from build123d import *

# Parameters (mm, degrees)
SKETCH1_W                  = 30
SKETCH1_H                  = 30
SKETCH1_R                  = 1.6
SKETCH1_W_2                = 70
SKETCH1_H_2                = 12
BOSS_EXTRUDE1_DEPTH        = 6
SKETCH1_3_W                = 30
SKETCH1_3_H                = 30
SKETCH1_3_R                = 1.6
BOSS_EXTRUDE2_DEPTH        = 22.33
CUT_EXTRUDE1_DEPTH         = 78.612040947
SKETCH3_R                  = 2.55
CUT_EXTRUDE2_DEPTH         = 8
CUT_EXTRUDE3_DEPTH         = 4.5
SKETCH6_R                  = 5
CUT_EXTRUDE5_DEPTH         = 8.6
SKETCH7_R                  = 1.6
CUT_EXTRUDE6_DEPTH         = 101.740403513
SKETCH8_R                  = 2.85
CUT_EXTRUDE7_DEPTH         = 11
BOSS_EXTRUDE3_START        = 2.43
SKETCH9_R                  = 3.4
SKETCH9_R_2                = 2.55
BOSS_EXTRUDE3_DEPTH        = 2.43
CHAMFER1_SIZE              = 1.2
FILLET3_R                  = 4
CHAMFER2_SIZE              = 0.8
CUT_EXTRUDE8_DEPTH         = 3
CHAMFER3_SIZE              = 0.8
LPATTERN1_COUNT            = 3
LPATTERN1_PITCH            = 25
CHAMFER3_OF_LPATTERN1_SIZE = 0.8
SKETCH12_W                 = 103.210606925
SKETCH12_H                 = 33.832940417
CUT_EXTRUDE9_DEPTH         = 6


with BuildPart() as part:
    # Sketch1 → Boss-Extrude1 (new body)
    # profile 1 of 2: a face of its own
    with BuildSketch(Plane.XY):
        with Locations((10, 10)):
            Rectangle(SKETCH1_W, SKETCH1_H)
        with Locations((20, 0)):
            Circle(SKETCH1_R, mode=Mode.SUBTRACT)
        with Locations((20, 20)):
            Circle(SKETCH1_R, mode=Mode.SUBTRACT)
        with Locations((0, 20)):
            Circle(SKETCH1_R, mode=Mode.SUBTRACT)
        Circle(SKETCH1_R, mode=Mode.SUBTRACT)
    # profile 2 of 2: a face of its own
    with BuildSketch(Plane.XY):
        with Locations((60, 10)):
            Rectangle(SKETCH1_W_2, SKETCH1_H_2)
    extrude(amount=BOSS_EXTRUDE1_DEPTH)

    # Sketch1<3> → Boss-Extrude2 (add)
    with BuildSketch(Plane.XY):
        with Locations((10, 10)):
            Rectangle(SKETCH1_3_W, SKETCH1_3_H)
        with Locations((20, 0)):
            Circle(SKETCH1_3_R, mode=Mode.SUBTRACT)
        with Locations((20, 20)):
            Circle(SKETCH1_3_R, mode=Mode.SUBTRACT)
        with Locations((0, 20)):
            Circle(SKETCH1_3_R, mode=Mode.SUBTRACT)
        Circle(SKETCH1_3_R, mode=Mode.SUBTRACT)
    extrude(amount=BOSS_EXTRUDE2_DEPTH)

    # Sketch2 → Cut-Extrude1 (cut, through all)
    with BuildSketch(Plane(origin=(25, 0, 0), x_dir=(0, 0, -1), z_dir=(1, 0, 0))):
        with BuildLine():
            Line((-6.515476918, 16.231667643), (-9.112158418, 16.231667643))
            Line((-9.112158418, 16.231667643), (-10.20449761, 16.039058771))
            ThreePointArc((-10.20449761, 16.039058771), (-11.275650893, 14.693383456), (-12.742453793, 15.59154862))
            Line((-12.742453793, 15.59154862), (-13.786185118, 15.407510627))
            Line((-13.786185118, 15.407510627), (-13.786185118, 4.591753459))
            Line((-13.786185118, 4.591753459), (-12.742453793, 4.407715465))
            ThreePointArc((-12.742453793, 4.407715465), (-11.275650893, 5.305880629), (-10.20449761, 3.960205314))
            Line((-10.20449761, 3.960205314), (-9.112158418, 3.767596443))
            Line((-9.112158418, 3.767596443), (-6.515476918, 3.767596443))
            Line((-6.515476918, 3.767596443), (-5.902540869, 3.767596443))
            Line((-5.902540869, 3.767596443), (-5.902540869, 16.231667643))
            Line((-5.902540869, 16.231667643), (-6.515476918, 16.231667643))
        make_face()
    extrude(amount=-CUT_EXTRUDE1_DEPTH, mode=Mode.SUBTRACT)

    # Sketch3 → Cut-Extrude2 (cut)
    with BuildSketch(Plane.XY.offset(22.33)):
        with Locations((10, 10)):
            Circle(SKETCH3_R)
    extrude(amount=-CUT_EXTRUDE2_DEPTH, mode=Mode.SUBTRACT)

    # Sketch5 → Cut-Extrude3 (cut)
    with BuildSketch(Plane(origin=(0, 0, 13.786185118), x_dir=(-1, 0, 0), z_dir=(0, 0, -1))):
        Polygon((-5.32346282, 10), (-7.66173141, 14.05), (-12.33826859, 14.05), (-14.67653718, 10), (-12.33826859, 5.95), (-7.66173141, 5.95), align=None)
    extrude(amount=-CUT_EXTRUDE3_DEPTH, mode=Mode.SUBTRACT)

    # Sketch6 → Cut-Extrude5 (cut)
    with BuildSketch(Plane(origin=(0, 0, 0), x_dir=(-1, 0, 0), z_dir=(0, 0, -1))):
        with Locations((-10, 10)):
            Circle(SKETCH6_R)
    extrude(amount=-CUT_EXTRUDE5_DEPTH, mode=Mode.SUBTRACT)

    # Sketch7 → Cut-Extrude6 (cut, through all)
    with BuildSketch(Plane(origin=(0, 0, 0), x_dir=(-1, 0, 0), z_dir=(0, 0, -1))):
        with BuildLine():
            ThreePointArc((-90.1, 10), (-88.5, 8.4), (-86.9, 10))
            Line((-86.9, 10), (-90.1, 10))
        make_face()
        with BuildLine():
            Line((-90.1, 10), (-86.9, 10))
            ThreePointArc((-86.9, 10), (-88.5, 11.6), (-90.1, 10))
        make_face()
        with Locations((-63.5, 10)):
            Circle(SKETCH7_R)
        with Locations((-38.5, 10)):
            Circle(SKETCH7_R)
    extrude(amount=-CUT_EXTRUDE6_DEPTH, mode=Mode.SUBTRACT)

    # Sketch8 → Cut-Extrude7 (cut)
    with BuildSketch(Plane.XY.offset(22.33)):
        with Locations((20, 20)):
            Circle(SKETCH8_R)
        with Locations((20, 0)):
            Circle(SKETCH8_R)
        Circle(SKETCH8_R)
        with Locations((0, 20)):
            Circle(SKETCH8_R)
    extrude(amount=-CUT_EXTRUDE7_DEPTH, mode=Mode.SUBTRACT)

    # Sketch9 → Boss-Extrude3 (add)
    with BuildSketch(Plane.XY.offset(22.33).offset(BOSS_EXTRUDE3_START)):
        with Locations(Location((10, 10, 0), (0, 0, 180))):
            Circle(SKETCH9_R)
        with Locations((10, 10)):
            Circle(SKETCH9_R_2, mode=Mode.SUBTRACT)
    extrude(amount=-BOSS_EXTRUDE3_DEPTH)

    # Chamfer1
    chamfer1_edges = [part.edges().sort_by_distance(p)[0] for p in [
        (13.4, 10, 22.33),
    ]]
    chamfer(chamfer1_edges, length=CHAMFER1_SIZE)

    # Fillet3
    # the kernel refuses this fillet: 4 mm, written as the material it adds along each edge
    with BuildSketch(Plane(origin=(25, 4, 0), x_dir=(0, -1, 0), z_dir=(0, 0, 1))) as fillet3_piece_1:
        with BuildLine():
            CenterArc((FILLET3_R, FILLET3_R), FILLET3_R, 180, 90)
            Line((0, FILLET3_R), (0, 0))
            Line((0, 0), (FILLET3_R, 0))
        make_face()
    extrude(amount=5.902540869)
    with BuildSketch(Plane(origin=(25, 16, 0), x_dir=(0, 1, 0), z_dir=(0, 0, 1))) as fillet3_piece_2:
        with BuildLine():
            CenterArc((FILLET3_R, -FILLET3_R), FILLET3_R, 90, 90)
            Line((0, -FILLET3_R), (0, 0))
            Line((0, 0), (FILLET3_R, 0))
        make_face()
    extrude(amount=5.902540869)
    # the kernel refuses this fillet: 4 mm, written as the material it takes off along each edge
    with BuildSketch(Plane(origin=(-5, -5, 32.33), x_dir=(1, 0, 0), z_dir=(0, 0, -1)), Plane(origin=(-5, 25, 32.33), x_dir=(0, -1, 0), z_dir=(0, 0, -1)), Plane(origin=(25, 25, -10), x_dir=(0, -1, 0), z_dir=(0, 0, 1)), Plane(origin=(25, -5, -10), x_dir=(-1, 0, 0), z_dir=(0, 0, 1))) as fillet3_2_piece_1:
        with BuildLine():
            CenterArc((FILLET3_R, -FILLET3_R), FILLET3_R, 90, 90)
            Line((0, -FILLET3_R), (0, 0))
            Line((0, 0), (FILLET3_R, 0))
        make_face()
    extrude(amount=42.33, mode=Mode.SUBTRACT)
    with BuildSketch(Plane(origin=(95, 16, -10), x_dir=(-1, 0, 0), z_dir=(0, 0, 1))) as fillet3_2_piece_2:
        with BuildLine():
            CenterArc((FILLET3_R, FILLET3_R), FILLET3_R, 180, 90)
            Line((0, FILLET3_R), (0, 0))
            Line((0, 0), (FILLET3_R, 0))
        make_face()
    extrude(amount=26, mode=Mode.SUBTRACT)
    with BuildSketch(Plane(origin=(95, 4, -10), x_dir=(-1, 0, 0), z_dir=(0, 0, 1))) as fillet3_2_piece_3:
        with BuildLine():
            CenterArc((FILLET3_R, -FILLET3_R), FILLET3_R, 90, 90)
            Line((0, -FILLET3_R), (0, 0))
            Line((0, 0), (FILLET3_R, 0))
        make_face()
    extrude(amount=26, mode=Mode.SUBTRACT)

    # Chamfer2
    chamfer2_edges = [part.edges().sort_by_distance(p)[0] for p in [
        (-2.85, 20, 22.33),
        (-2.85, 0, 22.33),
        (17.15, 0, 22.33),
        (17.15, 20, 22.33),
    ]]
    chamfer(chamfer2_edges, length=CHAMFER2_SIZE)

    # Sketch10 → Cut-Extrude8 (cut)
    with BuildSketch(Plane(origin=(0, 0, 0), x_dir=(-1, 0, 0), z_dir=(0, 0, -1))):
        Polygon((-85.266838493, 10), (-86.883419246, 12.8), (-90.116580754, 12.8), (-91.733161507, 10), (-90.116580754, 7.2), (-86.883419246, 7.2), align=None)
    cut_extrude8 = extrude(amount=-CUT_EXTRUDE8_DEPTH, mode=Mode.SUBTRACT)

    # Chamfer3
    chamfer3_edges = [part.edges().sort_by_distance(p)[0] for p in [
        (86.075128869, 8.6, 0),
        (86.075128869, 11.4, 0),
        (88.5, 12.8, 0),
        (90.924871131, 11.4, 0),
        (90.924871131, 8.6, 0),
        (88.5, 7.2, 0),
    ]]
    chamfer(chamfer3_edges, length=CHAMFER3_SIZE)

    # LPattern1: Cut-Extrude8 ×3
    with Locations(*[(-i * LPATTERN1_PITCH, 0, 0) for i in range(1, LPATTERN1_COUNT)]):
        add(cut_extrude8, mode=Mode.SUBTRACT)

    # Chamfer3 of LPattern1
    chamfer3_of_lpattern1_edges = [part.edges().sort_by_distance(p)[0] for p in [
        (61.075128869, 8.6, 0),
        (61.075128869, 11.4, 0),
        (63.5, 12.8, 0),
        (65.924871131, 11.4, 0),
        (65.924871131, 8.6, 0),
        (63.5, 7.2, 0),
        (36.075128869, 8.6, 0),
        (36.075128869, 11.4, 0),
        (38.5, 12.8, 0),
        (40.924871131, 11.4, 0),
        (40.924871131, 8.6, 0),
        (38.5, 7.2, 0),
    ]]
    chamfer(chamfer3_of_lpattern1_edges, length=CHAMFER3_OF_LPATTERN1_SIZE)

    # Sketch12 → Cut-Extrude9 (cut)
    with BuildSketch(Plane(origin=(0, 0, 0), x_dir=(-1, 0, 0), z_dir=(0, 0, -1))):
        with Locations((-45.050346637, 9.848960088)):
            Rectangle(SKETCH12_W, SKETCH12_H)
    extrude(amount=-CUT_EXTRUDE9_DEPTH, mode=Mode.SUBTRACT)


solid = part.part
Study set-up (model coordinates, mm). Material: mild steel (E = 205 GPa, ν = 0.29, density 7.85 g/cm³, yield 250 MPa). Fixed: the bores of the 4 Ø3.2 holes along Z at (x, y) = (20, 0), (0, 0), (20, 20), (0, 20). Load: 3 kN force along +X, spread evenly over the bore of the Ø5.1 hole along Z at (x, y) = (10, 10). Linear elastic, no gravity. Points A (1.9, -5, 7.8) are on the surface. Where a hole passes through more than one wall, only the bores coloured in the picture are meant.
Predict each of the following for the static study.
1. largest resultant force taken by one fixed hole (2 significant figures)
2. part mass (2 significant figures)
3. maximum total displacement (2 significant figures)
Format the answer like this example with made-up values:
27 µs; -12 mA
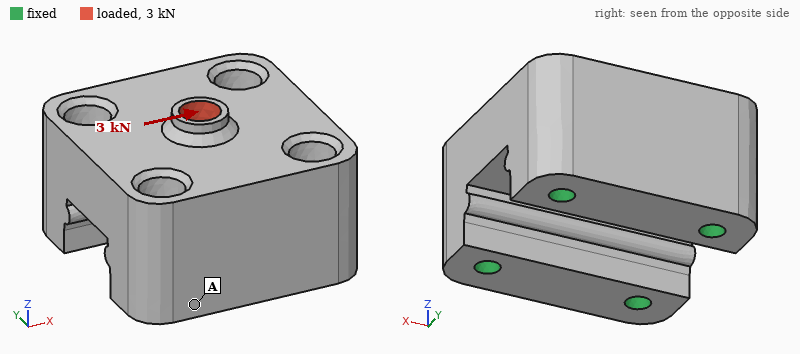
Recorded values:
1.2 kN; 80 g; 5.9 µm
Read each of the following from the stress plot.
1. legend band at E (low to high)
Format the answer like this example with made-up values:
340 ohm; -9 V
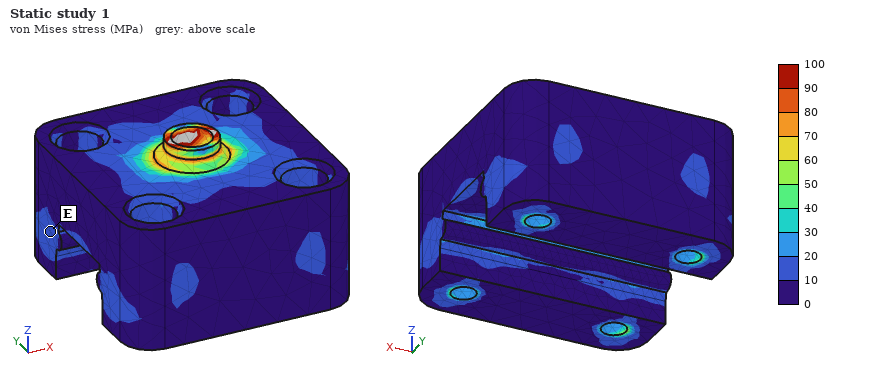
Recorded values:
10 to 20 MPa
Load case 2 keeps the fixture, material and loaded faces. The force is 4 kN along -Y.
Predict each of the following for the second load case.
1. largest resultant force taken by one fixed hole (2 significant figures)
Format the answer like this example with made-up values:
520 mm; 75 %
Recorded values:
1.4 kN
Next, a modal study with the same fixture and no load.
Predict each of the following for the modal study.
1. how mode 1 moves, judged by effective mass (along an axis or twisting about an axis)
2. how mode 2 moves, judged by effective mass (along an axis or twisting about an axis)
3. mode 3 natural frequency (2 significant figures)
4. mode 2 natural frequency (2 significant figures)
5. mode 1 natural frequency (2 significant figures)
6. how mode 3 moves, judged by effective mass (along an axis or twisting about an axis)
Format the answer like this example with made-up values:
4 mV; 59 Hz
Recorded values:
along Y; along X; 39 kHz; 31 kHz; 25 kHz; twisting about Z
